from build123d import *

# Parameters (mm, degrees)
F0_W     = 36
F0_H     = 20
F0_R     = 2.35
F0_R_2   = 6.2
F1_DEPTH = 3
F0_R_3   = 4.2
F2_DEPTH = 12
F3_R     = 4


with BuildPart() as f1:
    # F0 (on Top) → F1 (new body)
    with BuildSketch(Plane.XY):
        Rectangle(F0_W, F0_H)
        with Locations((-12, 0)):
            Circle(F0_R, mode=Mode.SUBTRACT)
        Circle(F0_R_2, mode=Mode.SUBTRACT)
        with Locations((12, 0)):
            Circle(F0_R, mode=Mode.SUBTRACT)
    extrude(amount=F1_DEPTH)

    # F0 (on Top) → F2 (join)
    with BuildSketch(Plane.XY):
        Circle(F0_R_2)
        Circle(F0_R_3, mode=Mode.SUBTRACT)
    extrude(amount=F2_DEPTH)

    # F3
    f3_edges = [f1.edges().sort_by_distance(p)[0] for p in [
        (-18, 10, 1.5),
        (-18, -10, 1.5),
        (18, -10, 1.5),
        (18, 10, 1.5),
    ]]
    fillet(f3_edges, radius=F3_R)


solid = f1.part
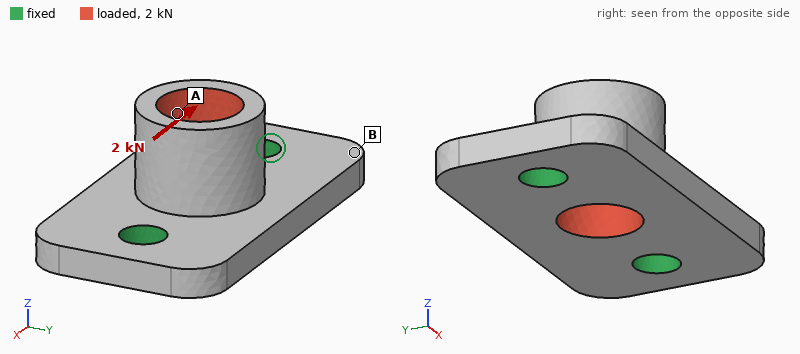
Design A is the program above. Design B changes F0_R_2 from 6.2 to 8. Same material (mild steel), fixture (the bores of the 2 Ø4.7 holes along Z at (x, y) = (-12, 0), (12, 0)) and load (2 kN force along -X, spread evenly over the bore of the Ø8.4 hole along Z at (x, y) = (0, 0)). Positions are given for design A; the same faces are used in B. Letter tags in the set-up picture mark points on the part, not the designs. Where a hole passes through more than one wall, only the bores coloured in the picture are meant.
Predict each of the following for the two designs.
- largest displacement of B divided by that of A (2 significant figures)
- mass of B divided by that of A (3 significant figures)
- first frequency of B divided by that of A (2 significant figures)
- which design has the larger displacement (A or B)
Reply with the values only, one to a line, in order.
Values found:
0.41
1.30
0.88
A
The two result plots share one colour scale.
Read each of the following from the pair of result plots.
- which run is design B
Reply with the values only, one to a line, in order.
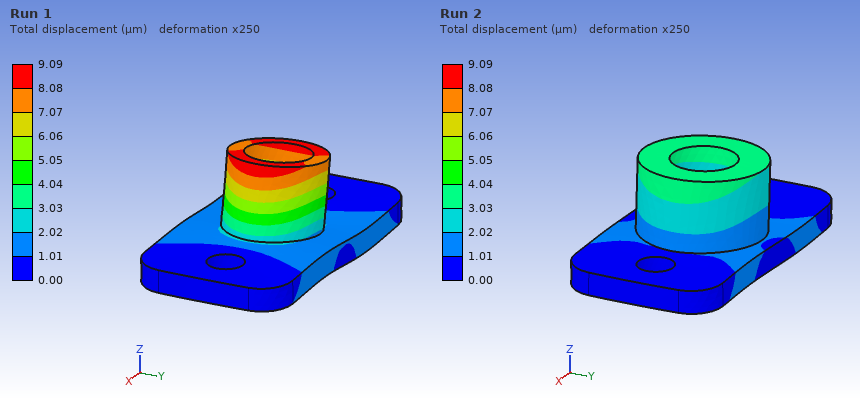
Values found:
Run 2
